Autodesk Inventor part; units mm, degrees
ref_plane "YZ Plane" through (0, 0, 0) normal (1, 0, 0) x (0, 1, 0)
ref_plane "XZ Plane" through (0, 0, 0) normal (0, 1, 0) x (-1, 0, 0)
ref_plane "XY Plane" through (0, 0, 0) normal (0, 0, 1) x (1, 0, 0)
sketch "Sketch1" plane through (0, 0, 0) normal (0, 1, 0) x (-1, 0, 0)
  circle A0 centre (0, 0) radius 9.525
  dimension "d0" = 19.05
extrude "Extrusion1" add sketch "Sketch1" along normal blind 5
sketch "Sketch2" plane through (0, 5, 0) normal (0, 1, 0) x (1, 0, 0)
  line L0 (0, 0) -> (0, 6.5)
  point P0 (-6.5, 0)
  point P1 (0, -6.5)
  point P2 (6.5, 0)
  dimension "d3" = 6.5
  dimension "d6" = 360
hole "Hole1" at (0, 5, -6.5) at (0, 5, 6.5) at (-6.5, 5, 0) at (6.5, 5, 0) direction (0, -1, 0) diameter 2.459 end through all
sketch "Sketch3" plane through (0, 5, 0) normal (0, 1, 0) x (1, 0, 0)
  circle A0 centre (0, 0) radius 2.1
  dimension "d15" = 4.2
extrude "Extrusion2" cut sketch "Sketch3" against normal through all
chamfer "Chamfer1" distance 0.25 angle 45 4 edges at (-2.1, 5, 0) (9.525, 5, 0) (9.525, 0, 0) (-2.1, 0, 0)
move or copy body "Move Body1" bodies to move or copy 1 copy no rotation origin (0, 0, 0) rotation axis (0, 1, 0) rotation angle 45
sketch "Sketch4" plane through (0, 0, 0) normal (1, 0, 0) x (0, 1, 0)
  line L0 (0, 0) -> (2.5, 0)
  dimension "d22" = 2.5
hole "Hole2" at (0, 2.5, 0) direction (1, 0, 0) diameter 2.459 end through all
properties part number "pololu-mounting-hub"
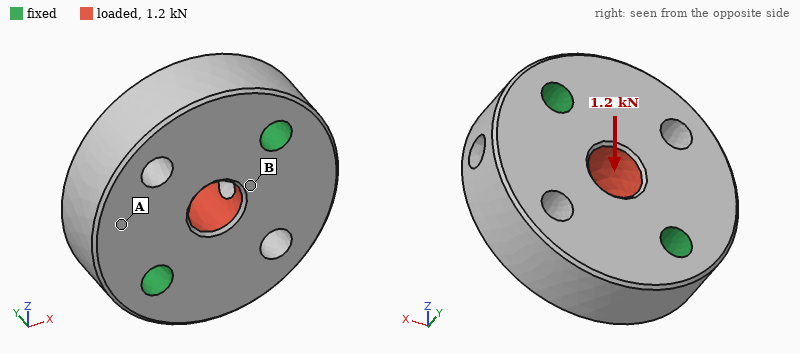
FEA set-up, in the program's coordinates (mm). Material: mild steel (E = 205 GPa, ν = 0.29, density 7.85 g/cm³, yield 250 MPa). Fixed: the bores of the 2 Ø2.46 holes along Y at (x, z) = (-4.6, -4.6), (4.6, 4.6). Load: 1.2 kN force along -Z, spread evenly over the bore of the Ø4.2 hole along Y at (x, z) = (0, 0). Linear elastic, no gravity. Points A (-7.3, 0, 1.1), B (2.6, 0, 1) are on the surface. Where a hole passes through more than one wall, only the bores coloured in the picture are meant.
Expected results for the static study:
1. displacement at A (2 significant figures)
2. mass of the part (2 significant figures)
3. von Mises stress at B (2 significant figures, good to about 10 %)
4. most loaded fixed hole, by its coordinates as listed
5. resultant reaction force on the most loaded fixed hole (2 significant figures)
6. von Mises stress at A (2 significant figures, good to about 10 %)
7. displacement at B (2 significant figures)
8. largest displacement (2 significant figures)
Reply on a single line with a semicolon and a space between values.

0.20 µm; 9.6 g; 23 MPa; (-4.6, -4.6); 660 N; 6.0 MPa; 0.46 µm; 0.81 µm
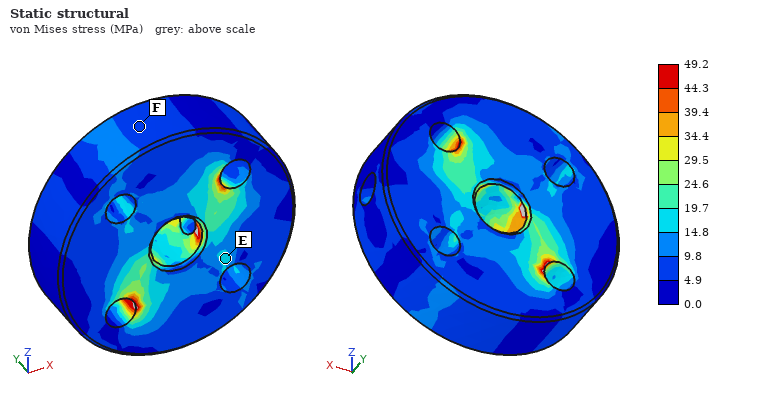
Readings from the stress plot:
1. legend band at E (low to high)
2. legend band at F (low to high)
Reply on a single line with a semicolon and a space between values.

14.8 to 19.7 MPa; 4.9 to 9.8 MPa
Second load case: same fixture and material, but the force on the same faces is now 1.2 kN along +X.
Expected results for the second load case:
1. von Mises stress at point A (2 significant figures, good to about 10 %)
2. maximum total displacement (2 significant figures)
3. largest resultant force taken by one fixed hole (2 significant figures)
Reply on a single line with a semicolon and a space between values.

6.1 MPa; 0.78 µm; 610 N
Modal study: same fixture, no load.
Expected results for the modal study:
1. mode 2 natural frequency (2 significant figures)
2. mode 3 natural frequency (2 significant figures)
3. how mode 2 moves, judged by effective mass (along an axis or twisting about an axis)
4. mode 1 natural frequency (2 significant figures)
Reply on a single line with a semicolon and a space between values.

46 kHz; 79 kHz; along Y; 40 kHz
